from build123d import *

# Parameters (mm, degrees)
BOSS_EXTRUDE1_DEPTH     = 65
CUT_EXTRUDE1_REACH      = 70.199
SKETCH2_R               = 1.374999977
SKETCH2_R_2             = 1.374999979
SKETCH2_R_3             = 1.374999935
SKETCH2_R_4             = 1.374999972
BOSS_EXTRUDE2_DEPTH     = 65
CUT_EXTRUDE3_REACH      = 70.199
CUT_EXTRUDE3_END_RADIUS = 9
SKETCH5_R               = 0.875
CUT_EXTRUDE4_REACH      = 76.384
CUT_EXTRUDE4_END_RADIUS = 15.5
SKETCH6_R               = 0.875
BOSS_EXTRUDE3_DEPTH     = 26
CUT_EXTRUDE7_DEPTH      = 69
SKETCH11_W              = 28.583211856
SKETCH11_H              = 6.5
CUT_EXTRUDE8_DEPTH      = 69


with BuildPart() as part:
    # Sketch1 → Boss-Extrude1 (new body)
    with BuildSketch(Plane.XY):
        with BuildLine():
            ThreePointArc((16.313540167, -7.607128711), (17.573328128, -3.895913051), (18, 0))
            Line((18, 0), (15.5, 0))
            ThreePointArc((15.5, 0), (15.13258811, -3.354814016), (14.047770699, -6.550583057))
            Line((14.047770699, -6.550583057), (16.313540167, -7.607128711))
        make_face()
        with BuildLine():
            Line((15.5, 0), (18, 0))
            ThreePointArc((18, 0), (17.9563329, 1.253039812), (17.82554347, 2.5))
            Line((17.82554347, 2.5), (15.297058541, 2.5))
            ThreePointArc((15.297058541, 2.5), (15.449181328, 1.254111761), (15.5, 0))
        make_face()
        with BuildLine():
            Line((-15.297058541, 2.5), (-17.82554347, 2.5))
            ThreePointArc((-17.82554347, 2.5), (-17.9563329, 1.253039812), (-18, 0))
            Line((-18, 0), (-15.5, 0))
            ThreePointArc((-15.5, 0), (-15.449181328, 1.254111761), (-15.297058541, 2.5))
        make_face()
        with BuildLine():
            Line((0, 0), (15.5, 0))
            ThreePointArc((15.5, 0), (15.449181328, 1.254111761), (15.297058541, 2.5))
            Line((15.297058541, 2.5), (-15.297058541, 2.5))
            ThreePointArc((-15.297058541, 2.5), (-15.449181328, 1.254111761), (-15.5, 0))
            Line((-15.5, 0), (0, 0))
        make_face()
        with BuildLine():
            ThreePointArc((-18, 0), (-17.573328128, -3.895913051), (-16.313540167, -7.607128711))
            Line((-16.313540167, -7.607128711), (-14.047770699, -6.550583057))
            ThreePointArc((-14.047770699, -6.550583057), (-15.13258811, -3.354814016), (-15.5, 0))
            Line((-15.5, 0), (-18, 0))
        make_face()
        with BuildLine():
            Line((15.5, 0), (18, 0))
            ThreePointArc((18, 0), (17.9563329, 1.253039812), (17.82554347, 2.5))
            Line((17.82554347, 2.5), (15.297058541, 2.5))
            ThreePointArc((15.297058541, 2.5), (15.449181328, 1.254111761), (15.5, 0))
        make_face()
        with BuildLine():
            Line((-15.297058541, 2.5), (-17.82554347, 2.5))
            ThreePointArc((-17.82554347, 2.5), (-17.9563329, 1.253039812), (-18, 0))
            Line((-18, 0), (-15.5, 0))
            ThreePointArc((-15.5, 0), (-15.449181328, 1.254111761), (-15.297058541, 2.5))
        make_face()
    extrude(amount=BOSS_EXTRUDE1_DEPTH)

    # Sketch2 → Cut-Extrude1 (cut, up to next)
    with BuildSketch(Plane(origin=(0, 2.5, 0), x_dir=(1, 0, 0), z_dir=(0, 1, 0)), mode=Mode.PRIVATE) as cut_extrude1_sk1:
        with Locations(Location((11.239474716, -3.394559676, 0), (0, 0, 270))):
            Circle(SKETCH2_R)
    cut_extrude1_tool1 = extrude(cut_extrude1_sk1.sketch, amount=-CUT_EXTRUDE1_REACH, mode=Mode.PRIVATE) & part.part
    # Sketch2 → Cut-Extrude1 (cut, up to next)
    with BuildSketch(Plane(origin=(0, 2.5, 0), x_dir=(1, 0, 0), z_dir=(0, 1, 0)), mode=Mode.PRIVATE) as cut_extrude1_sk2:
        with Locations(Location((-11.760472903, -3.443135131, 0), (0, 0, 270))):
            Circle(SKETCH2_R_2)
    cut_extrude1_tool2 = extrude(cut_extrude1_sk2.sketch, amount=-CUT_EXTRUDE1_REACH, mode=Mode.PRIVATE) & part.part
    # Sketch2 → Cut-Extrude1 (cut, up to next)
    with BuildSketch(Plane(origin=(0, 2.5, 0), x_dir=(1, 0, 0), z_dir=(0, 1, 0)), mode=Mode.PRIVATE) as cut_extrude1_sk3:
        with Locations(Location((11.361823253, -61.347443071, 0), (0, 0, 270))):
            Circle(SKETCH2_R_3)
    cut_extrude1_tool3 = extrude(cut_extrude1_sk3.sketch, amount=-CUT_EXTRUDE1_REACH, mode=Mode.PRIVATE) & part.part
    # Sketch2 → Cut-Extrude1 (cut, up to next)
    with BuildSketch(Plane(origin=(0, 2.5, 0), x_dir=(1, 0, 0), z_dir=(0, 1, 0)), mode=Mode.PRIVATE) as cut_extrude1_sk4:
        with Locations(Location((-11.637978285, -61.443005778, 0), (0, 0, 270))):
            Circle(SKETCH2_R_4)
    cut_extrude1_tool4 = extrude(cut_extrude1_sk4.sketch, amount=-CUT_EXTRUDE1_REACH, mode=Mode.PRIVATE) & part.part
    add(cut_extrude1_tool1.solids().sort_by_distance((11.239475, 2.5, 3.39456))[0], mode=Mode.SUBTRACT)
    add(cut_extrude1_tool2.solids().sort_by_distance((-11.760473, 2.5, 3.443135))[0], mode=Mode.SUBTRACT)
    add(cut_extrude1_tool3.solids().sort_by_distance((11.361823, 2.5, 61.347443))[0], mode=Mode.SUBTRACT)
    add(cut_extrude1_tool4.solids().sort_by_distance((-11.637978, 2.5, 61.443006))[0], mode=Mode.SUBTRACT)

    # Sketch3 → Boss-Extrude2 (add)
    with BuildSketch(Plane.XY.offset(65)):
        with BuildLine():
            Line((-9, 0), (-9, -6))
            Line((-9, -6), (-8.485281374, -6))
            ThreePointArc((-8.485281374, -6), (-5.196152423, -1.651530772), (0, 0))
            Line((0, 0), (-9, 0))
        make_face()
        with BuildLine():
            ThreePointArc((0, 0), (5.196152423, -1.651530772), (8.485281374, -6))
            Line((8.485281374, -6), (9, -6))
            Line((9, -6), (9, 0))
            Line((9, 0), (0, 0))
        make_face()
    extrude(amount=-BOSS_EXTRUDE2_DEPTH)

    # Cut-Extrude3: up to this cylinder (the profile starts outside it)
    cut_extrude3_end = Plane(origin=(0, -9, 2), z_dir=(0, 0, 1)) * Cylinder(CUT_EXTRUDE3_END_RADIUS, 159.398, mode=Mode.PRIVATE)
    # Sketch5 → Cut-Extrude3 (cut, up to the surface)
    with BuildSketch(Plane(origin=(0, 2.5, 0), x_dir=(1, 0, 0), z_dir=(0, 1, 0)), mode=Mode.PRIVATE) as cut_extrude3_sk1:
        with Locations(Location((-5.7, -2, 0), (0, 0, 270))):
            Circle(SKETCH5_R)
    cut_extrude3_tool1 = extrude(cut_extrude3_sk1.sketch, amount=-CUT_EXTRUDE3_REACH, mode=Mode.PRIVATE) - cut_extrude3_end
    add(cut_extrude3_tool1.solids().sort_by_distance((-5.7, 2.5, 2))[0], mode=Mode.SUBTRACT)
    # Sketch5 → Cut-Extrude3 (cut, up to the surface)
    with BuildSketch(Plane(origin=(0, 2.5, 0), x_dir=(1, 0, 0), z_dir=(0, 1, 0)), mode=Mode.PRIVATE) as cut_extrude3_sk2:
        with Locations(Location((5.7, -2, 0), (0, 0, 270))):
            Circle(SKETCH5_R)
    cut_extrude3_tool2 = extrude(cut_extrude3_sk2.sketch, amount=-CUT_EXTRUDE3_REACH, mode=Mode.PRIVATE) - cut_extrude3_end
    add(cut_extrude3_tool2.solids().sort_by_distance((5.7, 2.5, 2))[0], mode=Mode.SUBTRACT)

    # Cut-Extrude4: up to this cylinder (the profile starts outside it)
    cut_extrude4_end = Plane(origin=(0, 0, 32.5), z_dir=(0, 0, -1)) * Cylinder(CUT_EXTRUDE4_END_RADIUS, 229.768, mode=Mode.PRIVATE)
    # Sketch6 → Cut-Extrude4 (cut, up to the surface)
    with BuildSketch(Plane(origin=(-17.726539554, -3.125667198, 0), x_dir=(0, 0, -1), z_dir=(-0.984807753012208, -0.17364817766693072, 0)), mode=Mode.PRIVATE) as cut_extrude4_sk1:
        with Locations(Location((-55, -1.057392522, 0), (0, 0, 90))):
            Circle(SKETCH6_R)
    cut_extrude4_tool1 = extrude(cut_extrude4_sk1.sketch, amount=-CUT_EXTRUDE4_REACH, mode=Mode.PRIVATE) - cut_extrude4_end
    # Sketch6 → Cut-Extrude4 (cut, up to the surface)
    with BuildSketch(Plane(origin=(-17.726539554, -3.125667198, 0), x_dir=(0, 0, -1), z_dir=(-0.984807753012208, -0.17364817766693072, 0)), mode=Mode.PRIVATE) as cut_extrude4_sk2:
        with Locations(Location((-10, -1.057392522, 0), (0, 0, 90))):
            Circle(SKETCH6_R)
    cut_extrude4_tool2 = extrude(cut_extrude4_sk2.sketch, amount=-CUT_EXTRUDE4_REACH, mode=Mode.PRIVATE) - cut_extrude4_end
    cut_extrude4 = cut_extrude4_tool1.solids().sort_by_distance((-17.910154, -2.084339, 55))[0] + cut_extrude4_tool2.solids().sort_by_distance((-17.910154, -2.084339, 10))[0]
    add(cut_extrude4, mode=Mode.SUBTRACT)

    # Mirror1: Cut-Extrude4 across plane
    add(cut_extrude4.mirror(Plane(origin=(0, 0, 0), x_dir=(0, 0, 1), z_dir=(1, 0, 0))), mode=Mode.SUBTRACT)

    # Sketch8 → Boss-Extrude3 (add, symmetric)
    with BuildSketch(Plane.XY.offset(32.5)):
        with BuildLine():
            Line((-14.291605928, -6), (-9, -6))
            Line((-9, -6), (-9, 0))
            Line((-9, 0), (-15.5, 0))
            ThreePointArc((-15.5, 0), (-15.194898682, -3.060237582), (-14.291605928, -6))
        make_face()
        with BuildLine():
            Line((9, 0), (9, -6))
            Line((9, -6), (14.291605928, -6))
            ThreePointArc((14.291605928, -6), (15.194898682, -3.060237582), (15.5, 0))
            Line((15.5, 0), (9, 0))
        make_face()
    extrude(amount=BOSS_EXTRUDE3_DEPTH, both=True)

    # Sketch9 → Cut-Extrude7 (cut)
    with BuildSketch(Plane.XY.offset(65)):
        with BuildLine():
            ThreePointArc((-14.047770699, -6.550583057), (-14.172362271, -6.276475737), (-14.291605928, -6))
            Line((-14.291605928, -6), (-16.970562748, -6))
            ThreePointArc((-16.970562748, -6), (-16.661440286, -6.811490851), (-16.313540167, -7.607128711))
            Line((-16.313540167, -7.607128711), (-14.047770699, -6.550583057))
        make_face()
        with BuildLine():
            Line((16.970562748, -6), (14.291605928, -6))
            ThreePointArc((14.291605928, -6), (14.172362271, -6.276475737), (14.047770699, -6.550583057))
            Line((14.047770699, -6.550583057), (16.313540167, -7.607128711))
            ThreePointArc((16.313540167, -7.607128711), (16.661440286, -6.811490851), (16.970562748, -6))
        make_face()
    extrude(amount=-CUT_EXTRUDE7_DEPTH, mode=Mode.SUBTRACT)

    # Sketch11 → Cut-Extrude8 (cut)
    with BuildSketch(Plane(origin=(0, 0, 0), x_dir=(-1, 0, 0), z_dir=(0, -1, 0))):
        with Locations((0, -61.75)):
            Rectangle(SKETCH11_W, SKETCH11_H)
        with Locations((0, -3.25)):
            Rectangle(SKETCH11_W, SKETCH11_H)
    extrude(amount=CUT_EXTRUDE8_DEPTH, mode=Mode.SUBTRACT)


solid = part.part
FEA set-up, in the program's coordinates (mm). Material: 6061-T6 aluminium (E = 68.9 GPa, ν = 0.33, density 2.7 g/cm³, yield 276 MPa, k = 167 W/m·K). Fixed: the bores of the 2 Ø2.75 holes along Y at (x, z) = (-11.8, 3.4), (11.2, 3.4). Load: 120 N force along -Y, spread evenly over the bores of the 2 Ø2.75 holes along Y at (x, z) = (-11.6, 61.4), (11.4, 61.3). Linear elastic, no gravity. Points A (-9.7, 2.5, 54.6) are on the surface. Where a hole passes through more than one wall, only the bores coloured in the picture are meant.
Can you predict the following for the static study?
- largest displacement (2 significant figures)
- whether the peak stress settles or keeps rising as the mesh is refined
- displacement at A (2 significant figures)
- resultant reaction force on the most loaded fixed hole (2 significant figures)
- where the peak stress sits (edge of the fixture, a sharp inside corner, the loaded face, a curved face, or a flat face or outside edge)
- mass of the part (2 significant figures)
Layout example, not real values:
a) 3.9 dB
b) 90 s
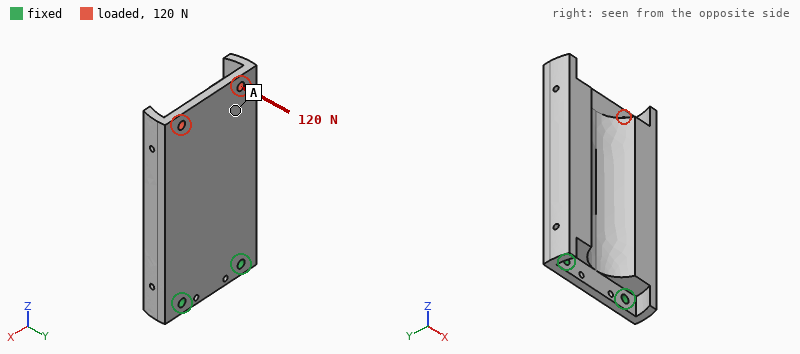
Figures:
a) 0.53 mm
b) keeps rising
c) 0.43 mm
d) 95 N
e) edge of the fixture
f) 36 g
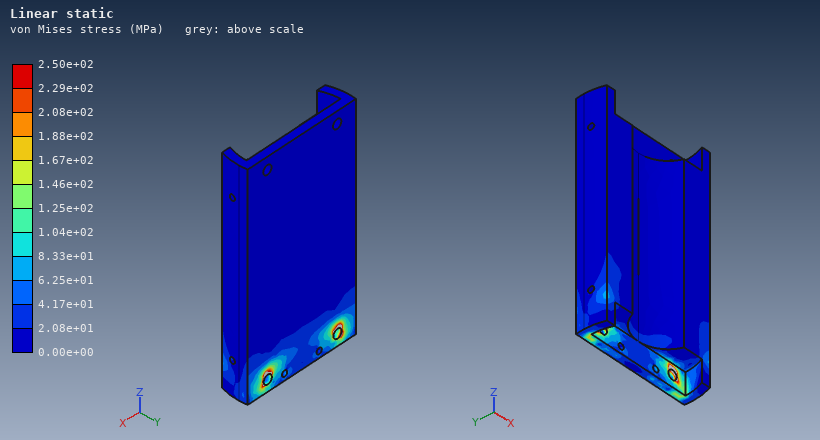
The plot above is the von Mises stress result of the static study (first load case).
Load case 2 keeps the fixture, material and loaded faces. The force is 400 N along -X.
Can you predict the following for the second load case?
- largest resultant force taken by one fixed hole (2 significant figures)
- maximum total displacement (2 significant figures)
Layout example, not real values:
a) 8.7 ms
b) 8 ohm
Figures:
a) 970 N
b) 53 µm
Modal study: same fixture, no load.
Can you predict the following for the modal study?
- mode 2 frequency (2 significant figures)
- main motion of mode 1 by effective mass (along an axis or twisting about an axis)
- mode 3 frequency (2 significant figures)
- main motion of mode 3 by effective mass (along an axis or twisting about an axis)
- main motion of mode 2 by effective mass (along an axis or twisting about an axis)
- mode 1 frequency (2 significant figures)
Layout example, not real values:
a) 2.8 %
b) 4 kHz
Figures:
a) 3400 Hz
b) along Y
c) 4500 Hz
d) along X
e) twisting about Z
f) 730 Hz
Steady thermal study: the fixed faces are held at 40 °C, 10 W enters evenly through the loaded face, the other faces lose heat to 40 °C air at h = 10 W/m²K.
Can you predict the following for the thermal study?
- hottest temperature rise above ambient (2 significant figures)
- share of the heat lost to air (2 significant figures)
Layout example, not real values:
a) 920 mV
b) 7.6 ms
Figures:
a) 22 K
b) 6.7 %
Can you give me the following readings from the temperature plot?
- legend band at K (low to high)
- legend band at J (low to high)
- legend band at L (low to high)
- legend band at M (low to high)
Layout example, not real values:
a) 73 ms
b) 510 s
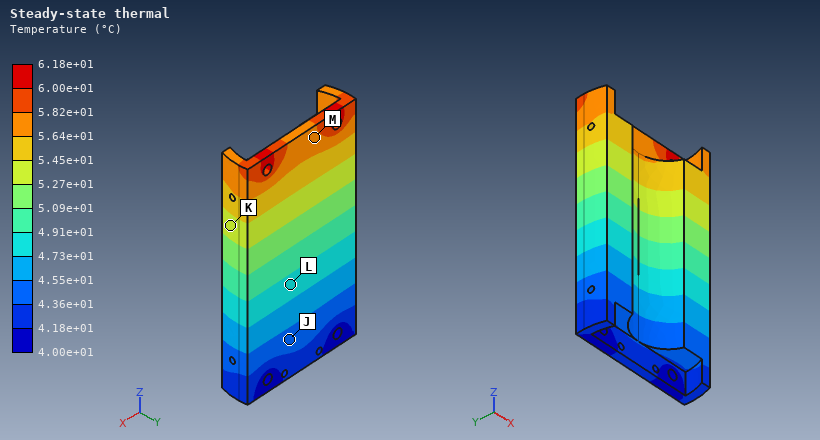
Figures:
a) 5.27e+01 to 5.45e+01 °C
b) 4.36e+01 to 4.55e+01 °C
c) 4.73e+01 to 4.91e+01 °C
d) 5.64e+01 to 5.82e+01 °C
